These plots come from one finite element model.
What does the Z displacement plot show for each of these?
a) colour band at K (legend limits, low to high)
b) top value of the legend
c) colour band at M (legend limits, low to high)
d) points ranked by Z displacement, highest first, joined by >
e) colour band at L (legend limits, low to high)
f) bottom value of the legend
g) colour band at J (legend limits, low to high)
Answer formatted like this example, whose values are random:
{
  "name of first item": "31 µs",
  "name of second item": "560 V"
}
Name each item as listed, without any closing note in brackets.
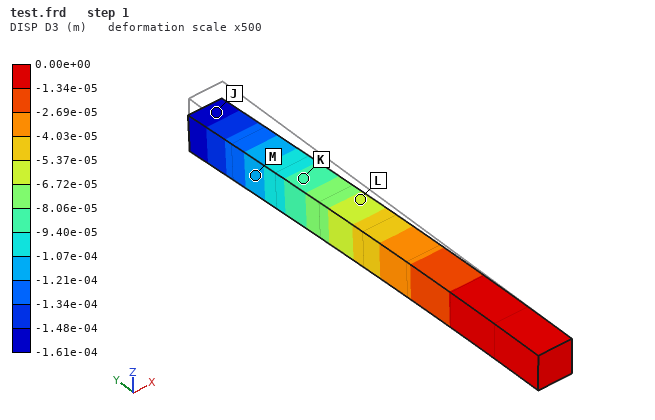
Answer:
{
  "colour band at K": "-9.40e-05 to -8.06e-05 m",
  "top value of the legend": "0.00e+00 m",
  "colour band at M": "-1.21e-04 to -1.07e-04 m",
  "points ranked by Z displacement, highest first, joined by >": "L > K > M > J",
  "colour band at L": "-6.72e-05 to -5.37e-05 m",
  "bottom value of the legend": "-1.61e-04 m",
  "colour band at J": "-1.61e-04 to -1.48e-04 m"
}
